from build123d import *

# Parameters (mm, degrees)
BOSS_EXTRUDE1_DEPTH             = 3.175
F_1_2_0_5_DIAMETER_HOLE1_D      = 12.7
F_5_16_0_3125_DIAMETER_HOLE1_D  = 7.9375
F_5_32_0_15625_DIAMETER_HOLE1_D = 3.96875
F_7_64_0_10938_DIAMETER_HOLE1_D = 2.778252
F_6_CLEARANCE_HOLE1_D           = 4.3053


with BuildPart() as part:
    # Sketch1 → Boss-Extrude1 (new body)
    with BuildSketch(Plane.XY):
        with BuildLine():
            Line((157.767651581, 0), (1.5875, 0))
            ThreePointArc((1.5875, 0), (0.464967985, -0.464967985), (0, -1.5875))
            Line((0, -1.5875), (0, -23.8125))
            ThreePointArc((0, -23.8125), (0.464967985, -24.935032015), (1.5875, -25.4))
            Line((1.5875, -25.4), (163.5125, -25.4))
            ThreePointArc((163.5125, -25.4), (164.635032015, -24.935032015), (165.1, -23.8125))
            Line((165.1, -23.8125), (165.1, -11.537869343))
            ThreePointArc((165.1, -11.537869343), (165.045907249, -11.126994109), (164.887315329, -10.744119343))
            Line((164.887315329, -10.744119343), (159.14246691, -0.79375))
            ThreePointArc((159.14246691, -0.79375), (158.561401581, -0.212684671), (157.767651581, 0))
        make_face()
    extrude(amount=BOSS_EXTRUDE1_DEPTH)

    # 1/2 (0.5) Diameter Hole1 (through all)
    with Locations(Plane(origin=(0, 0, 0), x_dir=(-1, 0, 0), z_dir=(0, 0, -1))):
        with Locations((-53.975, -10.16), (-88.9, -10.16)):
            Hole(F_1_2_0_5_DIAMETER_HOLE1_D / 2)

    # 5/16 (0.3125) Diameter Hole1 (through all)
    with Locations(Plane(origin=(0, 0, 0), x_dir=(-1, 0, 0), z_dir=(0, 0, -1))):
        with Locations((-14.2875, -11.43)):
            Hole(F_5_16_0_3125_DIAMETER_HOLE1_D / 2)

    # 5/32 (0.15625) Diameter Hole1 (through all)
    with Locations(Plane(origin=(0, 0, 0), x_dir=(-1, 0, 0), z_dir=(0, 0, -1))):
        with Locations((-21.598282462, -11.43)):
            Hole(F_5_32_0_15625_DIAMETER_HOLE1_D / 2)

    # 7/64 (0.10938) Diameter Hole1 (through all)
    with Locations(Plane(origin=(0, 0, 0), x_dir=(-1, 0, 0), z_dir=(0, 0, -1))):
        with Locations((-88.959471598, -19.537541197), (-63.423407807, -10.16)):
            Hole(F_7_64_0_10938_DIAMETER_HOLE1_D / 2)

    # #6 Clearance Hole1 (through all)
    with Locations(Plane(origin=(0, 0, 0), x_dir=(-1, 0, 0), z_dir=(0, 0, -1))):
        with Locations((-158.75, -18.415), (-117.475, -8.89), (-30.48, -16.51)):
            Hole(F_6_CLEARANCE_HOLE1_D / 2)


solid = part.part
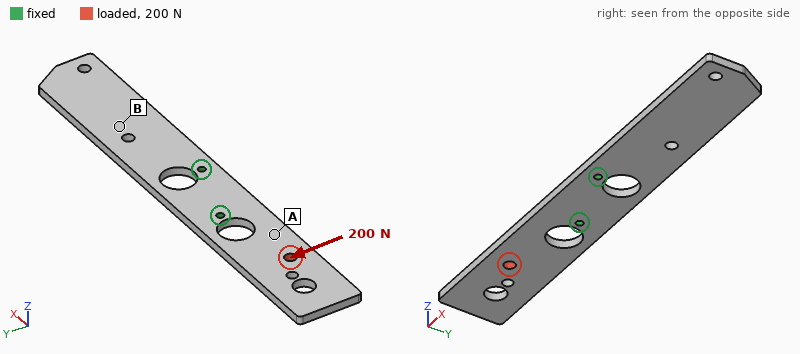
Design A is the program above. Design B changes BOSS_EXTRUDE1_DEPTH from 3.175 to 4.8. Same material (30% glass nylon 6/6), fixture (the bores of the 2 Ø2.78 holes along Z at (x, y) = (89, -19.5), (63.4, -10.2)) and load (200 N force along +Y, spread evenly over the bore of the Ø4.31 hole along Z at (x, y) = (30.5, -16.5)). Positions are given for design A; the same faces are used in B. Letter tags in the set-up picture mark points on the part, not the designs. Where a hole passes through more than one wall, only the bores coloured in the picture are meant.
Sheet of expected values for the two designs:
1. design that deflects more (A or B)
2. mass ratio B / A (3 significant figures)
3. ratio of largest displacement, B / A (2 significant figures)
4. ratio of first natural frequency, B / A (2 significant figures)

A
1.51
0.66
1.5
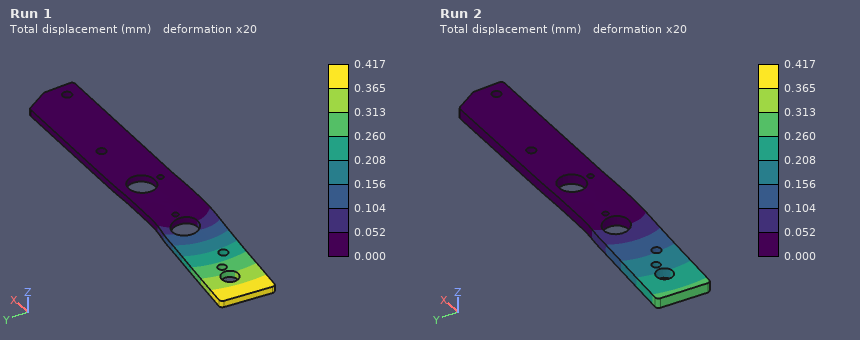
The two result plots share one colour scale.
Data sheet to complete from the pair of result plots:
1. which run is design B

Run 2
